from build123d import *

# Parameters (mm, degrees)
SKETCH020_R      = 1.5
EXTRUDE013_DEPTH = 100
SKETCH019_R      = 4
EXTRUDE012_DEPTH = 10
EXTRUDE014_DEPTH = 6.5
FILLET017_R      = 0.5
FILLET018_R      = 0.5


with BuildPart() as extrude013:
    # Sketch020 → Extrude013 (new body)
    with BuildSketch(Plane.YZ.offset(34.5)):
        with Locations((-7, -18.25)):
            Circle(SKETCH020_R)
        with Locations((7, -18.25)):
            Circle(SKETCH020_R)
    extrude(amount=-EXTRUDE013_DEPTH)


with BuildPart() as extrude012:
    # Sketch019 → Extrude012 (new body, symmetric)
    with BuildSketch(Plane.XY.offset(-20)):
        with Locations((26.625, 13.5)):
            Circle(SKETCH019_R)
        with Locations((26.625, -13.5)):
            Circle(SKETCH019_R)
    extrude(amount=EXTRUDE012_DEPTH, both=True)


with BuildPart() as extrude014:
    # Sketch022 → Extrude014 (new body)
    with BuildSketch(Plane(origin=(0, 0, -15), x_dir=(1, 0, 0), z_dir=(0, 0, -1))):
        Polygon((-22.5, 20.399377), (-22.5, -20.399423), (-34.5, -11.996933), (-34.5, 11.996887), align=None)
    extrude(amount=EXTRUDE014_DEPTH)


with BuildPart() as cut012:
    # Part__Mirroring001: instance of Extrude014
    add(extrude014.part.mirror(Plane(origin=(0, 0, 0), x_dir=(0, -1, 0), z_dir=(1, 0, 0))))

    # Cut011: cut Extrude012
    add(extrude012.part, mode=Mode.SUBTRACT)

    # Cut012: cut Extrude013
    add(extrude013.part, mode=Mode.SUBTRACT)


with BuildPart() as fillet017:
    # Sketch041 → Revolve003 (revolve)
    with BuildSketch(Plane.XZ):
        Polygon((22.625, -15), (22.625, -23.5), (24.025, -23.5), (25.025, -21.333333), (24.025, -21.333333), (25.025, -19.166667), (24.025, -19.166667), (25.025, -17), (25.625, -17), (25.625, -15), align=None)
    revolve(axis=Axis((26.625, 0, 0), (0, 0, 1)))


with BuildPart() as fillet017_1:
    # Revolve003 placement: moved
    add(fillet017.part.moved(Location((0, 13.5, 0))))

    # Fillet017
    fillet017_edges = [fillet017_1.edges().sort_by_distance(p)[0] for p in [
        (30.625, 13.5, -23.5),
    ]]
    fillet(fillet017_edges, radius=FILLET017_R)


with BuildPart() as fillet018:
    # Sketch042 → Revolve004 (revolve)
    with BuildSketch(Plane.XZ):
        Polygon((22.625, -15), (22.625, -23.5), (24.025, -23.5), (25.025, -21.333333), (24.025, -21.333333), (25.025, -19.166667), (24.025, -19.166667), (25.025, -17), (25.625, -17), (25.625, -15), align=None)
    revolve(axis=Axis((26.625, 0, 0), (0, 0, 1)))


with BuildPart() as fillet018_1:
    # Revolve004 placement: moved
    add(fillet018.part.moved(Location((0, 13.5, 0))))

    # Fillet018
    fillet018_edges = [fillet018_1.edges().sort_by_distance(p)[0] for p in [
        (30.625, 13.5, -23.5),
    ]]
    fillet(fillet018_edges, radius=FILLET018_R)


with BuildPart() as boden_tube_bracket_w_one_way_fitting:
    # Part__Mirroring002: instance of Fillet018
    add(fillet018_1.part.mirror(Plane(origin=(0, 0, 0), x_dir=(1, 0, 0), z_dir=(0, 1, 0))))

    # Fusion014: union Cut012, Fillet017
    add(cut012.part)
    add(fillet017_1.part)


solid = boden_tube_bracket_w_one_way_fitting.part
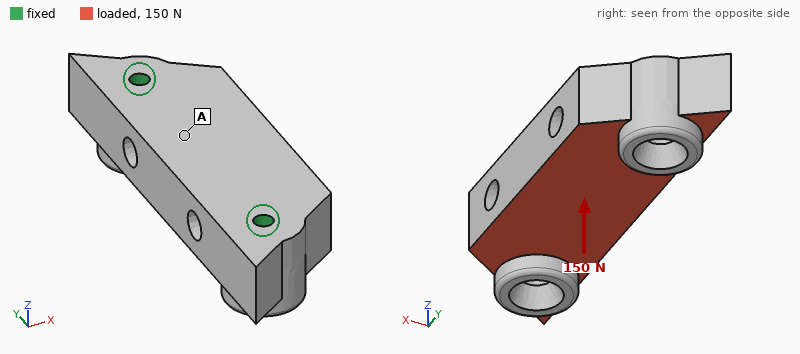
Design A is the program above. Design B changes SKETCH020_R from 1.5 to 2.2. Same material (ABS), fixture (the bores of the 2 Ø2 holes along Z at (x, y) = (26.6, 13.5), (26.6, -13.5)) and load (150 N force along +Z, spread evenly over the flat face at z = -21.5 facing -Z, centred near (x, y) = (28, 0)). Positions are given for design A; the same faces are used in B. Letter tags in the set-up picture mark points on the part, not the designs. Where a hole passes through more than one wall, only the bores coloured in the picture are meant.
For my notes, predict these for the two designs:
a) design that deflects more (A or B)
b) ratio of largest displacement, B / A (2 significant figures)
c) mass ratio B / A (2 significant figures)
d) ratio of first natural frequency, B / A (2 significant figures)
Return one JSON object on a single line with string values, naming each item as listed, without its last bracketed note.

{"design that deflects more": "B", "ratio of largest displacement, B / A": "1.2", "mass ratio B / A": "0.92", "ratio of first natural frequency, B / A": "1.0"}
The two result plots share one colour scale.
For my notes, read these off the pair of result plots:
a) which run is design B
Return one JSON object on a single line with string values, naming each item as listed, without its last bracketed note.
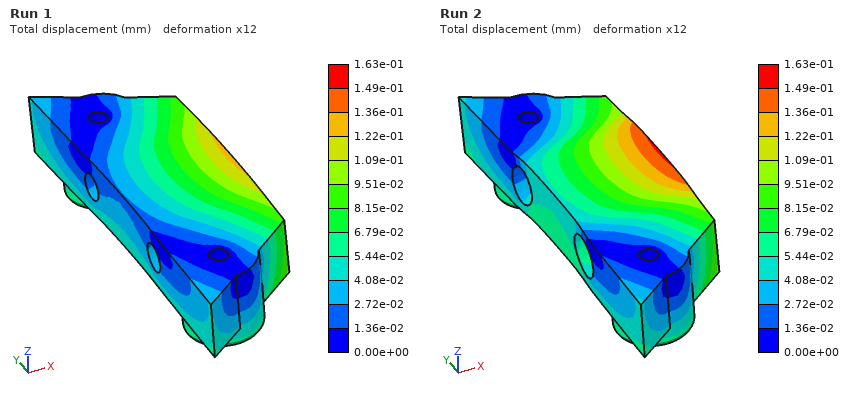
{"which run is design B": "Run 2"}
